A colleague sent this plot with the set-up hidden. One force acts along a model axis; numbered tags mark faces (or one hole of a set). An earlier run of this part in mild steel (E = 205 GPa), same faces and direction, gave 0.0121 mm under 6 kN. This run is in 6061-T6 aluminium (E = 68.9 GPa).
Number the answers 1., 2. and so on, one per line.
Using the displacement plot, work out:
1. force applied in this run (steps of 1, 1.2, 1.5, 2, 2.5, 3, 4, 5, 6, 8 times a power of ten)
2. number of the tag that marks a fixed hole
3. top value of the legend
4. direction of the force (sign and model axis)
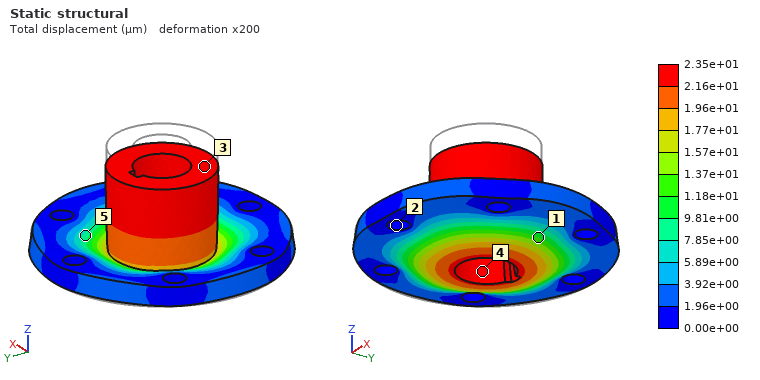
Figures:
1. 4 kN
2. 2
3. 2.35e+01 µm
4. -Z
